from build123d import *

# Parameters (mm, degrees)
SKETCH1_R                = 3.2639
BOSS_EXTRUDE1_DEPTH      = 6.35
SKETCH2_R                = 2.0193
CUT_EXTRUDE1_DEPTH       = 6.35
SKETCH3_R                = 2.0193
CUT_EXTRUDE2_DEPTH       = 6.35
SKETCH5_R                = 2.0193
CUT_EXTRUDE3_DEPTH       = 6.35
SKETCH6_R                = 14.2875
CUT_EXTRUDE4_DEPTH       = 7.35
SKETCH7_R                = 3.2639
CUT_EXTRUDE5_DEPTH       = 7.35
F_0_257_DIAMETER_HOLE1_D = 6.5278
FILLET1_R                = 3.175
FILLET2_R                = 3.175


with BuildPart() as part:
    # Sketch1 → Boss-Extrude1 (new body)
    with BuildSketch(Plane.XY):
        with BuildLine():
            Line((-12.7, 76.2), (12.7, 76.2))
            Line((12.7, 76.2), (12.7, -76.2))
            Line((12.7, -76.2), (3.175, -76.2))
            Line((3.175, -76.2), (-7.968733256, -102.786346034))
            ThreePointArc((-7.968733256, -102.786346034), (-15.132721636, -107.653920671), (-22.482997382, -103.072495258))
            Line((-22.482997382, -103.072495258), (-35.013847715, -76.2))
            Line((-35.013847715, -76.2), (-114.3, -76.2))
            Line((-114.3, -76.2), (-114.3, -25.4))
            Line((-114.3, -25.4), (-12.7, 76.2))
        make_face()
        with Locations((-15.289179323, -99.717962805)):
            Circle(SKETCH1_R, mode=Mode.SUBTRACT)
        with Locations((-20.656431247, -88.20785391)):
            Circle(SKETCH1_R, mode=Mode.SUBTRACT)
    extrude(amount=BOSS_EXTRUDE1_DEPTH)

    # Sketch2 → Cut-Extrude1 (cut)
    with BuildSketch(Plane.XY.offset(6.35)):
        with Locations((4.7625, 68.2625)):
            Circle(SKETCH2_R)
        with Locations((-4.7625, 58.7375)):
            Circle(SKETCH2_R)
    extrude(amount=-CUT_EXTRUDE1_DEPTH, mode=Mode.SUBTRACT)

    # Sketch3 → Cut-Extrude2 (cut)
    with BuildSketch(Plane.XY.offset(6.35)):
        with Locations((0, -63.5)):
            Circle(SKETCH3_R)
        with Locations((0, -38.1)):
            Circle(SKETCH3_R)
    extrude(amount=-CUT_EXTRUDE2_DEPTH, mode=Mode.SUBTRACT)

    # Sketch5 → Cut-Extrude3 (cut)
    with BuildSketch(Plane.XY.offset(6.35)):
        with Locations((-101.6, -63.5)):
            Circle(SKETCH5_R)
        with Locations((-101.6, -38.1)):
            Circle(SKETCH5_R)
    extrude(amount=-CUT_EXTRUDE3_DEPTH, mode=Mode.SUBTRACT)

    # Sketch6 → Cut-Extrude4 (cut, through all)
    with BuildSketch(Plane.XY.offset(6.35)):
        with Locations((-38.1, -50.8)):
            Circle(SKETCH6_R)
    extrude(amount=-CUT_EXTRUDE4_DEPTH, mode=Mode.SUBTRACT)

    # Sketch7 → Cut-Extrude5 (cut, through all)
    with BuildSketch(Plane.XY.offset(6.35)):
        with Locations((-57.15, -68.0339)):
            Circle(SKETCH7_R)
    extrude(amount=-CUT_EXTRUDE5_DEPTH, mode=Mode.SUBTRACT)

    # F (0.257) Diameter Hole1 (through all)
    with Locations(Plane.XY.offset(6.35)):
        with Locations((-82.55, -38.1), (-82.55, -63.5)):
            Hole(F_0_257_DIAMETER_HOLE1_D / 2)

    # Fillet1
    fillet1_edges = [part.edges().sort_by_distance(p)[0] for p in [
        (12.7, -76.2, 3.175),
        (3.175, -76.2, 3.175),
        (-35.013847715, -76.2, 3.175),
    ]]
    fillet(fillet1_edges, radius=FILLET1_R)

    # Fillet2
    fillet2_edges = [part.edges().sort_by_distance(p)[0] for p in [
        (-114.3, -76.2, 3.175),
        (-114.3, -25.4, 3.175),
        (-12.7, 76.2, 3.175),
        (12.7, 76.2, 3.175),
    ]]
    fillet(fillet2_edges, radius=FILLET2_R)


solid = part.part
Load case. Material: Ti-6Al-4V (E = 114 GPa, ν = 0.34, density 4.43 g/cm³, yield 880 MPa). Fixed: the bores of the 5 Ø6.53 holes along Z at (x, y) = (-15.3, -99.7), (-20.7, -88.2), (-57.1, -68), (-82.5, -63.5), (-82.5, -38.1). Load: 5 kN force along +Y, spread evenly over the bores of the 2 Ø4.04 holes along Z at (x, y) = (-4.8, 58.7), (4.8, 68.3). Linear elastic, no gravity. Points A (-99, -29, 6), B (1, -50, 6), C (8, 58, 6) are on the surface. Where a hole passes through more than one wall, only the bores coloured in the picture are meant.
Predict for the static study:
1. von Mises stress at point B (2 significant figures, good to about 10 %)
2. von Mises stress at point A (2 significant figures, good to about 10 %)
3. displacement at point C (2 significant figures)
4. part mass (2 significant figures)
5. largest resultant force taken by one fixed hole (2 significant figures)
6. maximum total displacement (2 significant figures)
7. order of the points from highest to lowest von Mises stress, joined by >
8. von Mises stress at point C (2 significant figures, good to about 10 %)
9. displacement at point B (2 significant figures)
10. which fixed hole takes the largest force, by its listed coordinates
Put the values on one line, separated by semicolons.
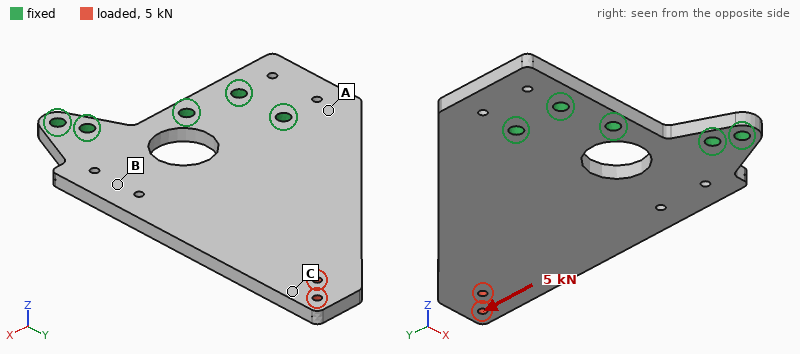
18 MPa; 6.3 MPa; 54 µm; 400 g; 3.0 kN; 64 µm; C > B > A; 30 MPa; 13 µm; (-20.7, -88.2)
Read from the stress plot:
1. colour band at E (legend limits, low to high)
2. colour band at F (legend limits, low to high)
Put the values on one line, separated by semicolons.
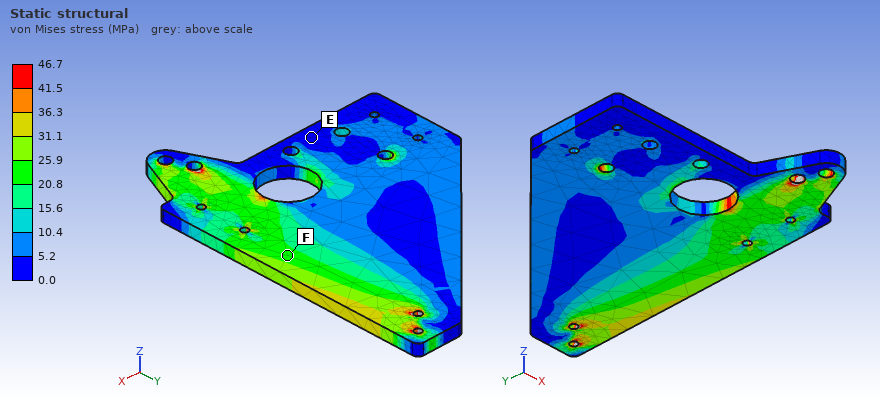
0.0 to 5.2 MPa; 20.8 to 25.9 MPa
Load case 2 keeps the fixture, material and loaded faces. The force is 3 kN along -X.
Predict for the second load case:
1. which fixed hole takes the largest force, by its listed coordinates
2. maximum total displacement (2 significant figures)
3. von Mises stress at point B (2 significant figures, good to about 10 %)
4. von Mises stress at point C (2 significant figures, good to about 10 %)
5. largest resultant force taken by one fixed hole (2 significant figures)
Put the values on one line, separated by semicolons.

(-82.5, -38.1); 74 µm; 14 MPa; 9.8 MPa; 5.1 kN
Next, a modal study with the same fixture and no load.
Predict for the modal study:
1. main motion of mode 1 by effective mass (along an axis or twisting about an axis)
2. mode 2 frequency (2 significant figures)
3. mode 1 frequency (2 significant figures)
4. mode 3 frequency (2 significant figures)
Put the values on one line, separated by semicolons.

along Z; 1400 Hz; 350 Hz; 1800 Hz
